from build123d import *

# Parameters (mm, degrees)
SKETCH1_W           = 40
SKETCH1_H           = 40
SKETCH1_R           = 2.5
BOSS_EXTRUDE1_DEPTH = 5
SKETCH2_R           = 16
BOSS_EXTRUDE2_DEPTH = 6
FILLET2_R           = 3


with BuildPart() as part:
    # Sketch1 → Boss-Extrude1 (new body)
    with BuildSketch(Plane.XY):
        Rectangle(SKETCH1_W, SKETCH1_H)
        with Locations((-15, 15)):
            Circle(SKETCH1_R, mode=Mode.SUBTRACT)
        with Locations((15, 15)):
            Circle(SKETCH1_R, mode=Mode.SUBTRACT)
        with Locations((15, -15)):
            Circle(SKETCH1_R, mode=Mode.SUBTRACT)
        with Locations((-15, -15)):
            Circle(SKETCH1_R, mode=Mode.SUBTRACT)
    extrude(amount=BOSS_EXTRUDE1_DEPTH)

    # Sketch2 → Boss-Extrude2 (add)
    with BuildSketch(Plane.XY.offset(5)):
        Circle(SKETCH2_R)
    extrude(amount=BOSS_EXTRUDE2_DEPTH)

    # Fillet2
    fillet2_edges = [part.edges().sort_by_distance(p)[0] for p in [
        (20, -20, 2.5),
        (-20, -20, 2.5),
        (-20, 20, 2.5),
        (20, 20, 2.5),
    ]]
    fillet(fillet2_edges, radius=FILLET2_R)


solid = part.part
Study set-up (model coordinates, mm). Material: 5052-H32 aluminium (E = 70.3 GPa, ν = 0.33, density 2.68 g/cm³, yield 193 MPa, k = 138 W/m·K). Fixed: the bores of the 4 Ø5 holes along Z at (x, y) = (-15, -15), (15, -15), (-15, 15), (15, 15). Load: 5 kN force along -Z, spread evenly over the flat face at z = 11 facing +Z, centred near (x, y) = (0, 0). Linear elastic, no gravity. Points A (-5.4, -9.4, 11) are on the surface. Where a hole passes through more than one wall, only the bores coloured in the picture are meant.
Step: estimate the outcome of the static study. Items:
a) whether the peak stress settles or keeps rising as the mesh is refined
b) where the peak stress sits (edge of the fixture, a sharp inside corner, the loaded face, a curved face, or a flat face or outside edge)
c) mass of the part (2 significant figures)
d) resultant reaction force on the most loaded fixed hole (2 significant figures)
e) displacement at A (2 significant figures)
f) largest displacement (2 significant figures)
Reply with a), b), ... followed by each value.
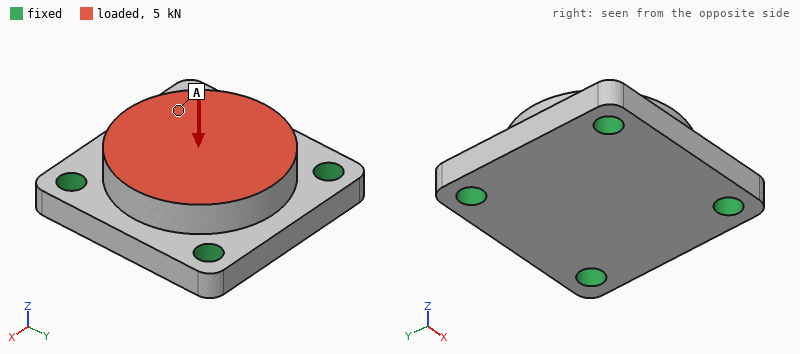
a) keeps rising
b) edge of the fixture
c) 33 g
d) 1.4 kN
e) 9.4 µm
f) 11 µm
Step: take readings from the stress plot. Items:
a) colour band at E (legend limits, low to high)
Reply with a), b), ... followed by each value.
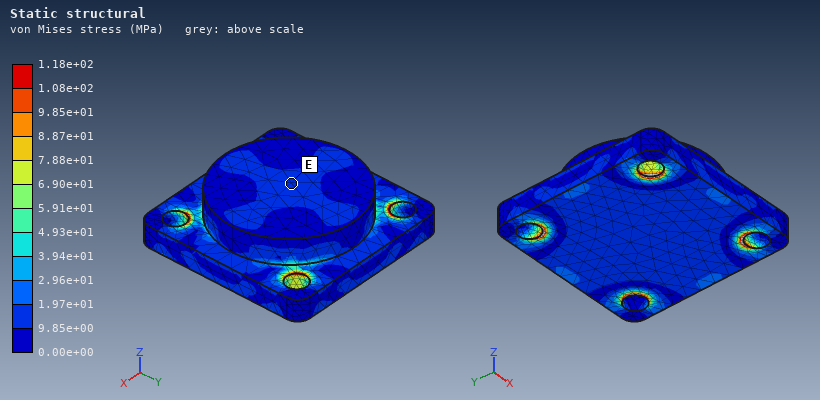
a) 9.85e+00 to 1.97e+01 MPa
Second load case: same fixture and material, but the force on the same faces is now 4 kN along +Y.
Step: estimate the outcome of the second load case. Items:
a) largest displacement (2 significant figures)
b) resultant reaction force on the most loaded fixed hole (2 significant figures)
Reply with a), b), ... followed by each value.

a) 9.1 µm
b) 1.2 kN
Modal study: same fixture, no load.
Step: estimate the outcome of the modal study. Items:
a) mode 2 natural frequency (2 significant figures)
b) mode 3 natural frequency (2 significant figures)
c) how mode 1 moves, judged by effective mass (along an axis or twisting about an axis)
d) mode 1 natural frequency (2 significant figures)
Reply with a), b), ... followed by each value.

a) 30 kHz
b) 30 kHz
c) along Z
d) 22 kHz
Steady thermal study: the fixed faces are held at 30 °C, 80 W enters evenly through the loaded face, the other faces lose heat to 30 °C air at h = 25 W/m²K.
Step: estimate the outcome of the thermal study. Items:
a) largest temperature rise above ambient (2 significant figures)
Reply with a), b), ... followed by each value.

a) 20 K
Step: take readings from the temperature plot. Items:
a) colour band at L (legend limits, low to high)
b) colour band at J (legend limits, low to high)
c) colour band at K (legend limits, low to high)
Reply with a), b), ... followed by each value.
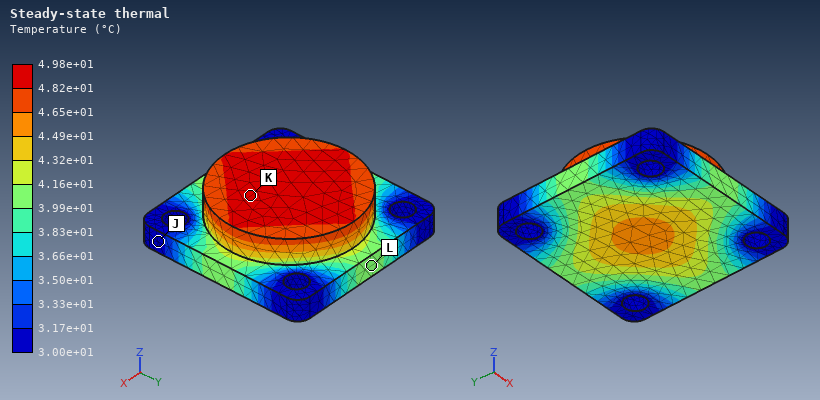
a) 3.99e+01 to 4.16e+01 °C
b) 3.00e+01 to 3.17e+01 °C
c) 4.82e+01 to 4.98e+01 °C
